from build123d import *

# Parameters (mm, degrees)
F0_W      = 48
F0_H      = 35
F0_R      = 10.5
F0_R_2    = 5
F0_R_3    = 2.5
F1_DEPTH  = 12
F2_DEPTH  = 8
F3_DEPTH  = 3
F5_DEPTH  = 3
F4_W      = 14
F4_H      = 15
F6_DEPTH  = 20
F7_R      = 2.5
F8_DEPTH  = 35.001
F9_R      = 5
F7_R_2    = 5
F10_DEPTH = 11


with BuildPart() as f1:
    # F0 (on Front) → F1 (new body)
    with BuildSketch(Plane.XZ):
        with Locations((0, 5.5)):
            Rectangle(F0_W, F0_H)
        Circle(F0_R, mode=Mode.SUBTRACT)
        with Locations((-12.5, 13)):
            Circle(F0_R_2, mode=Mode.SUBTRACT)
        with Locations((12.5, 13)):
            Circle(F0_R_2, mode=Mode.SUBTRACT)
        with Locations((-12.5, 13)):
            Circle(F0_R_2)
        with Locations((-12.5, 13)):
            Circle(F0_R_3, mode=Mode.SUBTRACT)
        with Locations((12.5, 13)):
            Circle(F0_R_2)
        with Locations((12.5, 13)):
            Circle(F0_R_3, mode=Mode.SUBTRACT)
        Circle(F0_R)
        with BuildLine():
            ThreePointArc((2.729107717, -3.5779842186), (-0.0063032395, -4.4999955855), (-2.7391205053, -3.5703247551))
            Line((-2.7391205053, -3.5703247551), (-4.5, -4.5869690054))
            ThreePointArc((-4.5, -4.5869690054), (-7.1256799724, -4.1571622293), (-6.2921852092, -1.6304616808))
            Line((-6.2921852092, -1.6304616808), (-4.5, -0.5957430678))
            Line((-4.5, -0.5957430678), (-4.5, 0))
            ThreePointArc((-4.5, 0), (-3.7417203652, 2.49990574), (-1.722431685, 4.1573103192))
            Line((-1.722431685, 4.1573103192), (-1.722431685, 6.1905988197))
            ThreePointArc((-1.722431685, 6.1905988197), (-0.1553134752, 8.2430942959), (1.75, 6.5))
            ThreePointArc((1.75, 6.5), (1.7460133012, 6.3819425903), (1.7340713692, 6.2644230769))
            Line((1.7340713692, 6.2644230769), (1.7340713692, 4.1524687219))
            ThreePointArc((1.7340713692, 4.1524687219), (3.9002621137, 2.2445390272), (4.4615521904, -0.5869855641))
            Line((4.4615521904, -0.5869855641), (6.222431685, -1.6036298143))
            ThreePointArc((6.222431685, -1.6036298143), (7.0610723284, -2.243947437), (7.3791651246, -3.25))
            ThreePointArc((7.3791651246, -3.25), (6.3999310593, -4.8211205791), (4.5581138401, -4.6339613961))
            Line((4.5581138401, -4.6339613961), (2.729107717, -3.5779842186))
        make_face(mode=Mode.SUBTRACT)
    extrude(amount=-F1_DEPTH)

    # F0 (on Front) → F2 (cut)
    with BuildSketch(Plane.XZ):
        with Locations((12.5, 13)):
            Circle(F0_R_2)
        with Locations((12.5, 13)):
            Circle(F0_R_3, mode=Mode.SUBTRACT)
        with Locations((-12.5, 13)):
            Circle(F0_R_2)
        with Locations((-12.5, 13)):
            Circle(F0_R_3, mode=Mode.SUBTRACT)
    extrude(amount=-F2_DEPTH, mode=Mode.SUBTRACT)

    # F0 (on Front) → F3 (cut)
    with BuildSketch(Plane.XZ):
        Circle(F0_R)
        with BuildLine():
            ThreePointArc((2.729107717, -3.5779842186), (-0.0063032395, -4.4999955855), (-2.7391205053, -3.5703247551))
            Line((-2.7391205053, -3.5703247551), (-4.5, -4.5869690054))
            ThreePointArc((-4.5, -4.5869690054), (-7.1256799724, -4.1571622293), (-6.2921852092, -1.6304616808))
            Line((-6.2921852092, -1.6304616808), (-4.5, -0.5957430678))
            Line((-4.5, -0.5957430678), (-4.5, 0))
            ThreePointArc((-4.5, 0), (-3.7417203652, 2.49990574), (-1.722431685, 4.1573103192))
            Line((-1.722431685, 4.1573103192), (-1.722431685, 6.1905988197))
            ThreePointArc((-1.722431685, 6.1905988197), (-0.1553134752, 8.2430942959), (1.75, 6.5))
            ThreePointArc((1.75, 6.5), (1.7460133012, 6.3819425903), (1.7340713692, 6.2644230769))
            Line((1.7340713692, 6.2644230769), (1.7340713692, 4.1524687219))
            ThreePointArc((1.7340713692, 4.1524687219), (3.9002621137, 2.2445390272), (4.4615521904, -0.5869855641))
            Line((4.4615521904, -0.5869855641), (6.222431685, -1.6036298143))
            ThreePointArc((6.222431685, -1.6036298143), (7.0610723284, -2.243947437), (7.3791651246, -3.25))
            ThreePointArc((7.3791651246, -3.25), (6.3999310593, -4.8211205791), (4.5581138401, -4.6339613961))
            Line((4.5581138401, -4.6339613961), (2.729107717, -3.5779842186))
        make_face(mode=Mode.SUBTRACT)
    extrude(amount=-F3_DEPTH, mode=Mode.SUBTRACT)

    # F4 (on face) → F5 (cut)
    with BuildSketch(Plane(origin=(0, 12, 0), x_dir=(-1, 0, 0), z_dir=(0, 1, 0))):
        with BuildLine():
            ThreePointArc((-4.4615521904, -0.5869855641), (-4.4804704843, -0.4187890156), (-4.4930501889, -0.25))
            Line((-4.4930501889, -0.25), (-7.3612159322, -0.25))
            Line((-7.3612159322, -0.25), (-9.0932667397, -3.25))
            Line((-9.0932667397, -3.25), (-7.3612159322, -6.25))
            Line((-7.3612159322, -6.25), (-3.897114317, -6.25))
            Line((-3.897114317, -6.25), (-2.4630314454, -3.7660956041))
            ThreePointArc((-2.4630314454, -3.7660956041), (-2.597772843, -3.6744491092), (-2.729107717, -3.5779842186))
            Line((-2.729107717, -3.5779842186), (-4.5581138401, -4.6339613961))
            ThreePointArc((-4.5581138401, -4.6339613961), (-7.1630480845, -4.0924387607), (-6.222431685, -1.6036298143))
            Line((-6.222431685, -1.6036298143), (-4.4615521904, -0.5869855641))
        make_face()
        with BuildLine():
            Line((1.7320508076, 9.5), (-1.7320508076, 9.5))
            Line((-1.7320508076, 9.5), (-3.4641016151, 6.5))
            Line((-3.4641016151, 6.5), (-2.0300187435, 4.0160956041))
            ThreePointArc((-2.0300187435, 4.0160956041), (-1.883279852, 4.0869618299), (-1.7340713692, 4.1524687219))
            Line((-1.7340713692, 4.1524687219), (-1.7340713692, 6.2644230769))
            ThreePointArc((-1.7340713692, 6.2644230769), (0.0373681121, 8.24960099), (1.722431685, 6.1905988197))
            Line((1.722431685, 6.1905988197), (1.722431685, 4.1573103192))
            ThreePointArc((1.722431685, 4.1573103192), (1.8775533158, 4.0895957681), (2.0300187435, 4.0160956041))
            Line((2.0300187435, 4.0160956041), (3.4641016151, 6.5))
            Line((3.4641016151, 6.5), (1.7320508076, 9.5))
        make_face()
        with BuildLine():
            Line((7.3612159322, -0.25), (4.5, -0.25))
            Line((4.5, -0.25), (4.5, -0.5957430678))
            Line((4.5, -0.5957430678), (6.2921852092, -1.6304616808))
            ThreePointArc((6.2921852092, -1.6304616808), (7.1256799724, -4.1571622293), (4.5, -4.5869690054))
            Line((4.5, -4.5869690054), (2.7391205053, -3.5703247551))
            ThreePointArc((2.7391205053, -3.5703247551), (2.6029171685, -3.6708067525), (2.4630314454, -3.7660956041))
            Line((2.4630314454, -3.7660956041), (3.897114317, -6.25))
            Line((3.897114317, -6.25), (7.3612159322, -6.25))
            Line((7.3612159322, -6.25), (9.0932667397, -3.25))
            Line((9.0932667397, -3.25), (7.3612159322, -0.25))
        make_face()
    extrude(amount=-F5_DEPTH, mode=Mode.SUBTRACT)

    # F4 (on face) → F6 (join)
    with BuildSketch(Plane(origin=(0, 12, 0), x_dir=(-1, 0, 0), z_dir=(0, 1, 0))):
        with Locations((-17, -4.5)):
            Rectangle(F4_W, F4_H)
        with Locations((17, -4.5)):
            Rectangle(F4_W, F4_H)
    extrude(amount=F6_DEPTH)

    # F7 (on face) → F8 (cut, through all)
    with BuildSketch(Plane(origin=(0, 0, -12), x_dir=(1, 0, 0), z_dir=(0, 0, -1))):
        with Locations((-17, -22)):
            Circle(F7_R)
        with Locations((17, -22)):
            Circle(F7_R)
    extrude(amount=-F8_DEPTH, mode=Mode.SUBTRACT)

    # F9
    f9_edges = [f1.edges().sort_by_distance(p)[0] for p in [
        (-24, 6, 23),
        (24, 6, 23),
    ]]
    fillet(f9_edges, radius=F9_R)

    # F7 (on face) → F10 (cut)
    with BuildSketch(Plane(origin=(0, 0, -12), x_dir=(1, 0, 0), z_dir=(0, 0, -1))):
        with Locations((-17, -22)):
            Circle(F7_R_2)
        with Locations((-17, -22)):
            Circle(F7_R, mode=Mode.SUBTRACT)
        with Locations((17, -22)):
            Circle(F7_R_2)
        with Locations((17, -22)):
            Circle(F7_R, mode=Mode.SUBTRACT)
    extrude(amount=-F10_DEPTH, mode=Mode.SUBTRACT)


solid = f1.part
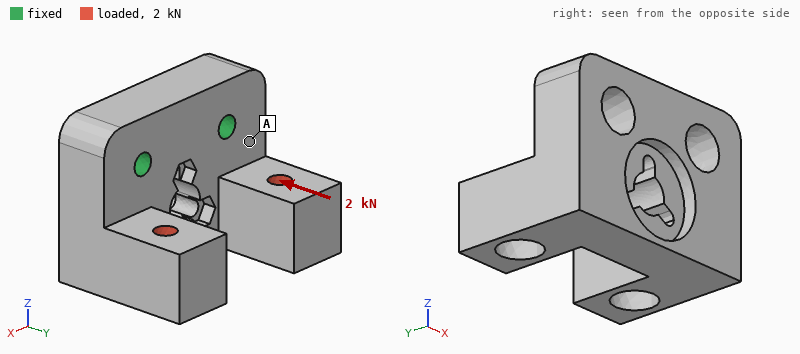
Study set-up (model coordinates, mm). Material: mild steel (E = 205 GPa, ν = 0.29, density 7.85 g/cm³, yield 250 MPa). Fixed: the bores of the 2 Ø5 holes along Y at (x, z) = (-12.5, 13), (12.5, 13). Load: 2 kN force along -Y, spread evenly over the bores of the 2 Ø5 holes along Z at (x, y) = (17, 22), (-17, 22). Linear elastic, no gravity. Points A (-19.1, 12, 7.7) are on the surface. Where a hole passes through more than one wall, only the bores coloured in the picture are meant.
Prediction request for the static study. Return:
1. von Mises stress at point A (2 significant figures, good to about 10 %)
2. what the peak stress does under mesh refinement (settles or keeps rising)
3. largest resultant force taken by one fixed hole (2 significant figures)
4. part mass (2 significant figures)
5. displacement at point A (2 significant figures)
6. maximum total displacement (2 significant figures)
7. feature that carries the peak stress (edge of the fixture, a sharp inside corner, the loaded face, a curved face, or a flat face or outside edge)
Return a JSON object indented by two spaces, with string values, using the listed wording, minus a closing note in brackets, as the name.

{
  "von Mises stress at point A": "18 MPa",
  "what the peak stress does under mesh refinement": "keeps rising",
  "largest resultant force taken by one fixed hole": "1.0 kN",
  "part mass": "180 g",
  "displacement at point A": "5.4 µm",
  "maximum total displacement": "29 µm",
  "feature that carries the peak stress": "edge of the fixture"
}
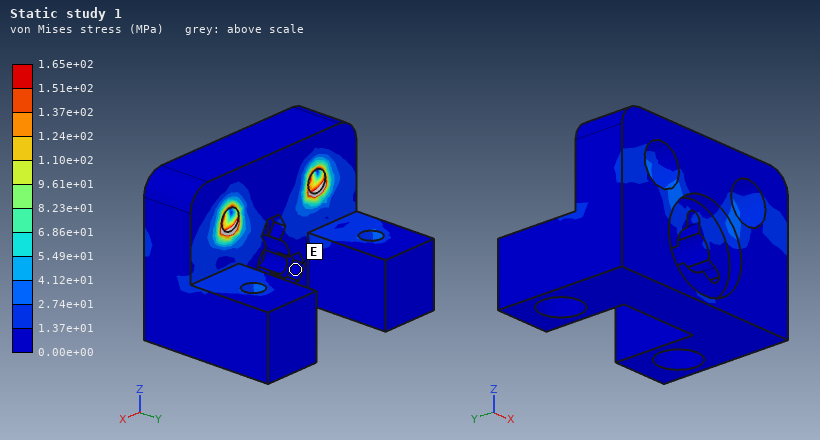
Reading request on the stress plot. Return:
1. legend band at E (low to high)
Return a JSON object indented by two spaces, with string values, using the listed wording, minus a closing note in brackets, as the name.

{
  "legend band at E": "0.00e+00 to 1.37e+01 MPa"
}
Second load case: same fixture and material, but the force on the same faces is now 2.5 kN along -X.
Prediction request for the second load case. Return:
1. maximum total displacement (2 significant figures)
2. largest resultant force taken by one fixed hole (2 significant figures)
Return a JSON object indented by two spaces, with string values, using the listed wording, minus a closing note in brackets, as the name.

{
  "maximum total displacement": "28 µm",
  "largest resultant force taken by one fixed hole": "1.8 kN"
}
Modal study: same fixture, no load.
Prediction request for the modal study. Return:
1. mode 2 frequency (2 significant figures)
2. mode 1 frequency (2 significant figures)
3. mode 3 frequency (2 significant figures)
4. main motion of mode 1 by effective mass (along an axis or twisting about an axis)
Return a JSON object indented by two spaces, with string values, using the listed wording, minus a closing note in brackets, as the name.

{
  "mode 2 frequency": "5900 Hz",
  "mode 1 frequency": "3500 Hz",
  "mode 3 frequency": "8300 Hz",
  "main motion of mode 1 by effective mass": "along Y"
}
